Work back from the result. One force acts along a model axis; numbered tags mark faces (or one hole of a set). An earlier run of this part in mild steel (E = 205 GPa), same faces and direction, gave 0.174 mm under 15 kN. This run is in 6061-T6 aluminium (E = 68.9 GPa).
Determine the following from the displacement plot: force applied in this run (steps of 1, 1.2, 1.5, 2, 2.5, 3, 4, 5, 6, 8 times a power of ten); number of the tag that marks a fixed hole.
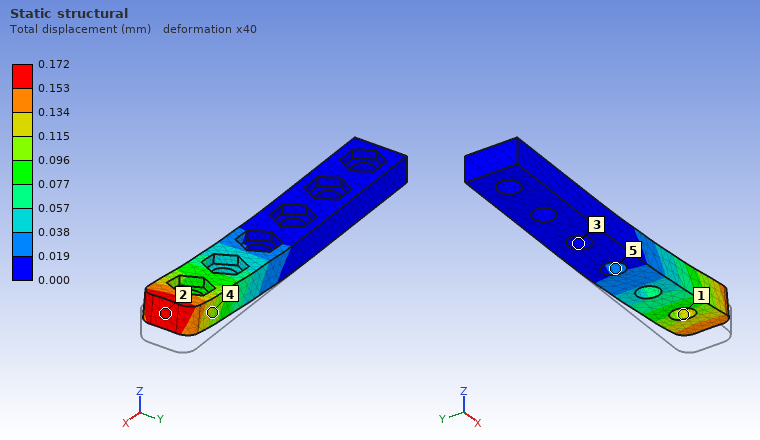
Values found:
5 kN
3
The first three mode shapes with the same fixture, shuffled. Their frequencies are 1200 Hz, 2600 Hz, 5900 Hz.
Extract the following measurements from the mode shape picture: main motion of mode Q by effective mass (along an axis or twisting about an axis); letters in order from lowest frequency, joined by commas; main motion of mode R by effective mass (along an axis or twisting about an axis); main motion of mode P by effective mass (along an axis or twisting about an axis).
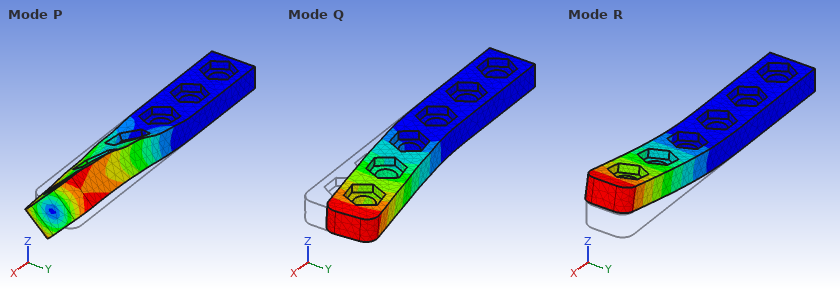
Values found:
along Y
R, Q, P
along Z
twisting about X
